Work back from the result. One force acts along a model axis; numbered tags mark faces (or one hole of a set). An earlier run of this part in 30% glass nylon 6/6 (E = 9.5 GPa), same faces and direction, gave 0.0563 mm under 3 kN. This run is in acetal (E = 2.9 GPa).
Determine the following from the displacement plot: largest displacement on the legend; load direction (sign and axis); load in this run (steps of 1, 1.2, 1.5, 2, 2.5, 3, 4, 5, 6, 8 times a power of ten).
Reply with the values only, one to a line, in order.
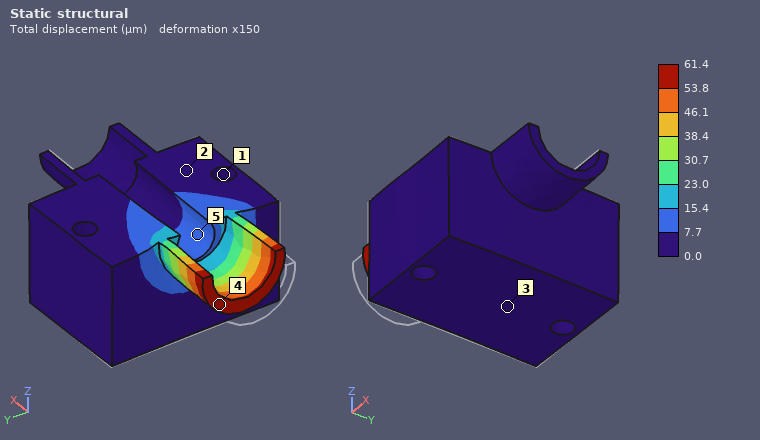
61.4 µm
+X
1 kN
